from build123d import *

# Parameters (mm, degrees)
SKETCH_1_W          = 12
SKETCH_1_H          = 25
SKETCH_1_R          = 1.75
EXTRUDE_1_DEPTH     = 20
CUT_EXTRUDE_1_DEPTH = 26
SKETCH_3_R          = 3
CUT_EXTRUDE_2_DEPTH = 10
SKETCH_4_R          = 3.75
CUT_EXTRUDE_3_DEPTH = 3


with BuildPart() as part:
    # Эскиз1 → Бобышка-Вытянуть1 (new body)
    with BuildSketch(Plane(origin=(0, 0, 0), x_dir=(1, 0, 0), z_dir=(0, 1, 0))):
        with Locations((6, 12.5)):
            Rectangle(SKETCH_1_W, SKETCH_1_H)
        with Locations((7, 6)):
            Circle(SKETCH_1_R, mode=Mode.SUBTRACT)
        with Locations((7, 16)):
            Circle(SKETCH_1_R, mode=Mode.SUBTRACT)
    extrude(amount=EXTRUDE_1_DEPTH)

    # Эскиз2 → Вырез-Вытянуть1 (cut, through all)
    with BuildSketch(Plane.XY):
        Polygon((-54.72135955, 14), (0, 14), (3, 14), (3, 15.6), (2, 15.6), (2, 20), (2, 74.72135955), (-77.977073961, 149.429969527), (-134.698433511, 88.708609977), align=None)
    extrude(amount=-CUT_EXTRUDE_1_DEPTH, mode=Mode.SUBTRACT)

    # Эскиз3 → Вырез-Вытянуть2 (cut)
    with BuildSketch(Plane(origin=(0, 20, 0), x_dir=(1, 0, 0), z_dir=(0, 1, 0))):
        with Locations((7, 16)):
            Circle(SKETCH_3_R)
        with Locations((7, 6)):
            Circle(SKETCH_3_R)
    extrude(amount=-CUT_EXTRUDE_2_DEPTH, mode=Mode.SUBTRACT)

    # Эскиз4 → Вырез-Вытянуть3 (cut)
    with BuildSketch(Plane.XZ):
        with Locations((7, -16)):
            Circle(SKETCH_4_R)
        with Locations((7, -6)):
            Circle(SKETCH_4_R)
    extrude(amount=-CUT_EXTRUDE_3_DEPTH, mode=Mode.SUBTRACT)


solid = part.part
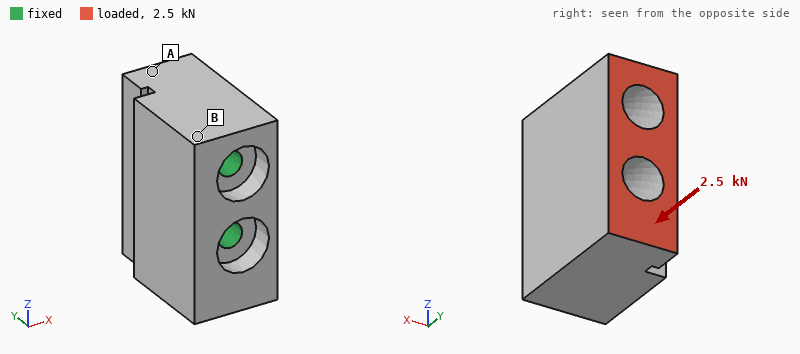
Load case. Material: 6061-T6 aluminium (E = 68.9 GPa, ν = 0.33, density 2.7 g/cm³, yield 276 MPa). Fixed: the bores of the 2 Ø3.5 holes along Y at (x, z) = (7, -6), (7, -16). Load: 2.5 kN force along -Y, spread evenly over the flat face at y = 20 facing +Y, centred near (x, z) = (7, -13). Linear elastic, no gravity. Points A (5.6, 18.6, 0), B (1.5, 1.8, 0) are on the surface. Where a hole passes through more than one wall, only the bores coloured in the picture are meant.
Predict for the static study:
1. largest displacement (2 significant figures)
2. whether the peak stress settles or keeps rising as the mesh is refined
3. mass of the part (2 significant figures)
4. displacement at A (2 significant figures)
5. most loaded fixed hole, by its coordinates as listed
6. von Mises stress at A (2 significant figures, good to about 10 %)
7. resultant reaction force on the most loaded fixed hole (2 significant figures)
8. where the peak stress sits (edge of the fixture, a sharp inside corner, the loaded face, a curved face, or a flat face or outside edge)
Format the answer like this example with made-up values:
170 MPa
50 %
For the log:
6.5 µm
keeps rising
13 g
2.8 µm
(7, -16)
14 MPa
1.6 kN
edge of the fixture
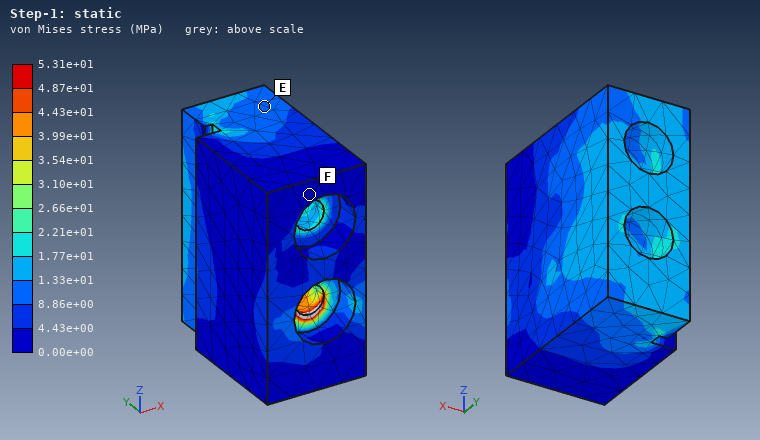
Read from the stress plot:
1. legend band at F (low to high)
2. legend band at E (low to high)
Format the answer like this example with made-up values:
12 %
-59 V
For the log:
0.00e+00 to 4.43e+00 MPa
8.86e+00 to 1.33e+01 MPa
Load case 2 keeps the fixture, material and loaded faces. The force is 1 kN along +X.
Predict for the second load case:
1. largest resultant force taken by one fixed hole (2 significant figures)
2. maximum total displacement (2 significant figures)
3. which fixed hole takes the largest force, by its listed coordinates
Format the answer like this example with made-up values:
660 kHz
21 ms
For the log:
640 N
18 µm
(7, -16)
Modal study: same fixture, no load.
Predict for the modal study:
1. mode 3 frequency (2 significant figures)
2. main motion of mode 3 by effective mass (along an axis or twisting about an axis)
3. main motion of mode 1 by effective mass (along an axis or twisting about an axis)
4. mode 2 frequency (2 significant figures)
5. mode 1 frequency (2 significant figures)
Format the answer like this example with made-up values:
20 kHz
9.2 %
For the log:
34 kHz
twisting about Y
along X
31 kHz
25 kHz
